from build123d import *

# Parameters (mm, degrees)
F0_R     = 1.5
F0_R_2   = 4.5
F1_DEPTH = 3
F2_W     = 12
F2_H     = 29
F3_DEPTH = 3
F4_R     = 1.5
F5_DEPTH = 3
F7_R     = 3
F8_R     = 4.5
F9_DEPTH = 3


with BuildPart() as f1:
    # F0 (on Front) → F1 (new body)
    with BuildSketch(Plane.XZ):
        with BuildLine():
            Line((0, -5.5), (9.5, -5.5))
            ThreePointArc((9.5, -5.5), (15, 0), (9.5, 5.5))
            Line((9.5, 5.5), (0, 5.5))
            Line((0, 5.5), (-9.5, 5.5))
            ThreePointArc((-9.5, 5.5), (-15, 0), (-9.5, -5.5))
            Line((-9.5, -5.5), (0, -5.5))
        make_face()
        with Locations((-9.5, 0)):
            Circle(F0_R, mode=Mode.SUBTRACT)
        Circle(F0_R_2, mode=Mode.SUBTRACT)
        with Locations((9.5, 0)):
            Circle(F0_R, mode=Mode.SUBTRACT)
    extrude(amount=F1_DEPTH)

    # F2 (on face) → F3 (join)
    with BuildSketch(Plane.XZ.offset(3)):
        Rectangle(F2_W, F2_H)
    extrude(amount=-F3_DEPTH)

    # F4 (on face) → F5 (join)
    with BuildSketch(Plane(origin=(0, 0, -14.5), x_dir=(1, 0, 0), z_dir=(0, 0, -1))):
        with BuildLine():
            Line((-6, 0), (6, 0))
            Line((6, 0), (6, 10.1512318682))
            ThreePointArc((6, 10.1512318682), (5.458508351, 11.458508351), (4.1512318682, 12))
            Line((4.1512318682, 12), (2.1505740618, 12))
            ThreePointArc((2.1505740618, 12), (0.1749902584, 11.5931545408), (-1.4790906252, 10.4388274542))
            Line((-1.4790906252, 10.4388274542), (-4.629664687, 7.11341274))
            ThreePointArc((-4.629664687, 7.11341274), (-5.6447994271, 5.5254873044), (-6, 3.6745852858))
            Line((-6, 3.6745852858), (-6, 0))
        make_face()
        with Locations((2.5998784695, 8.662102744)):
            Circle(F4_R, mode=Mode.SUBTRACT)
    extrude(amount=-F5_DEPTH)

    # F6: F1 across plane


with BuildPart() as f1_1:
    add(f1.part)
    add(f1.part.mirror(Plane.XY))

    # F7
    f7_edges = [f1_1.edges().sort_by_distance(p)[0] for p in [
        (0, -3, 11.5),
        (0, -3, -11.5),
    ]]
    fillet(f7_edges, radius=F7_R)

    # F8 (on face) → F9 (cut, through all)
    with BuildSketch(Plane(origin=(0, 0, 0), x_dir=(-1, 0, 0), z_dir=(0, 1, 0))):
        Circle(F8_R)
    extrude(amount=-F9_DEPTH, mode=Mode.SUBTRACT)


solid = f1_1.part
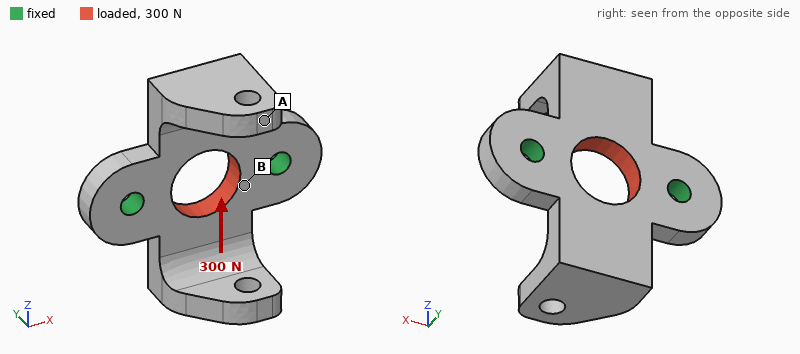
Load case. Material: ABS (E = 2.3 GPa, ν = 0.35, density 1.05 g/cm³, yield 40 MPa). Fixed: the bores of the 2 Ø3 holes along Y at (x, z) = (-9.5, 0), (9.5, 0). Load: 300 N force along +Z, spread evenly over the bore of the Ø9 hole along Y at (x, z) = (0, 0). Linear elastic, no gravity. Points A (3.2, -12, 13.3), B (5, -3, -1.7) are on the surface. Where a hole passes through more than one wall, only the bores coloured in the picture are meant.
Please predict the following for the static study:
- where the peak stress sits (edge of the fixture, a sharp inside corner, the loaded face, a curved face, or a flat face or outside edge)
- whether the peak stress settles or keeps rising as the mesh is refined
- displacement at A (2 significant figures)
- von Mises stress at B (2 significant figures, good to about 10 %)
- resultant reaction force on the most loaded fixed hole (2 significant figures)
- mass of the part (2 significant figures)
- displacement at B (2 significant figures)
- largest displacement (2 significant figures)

edge of the fixture
keeps rising
33 µm
6.4 MPa
150 N
1.9 g
29 µm
40 µm
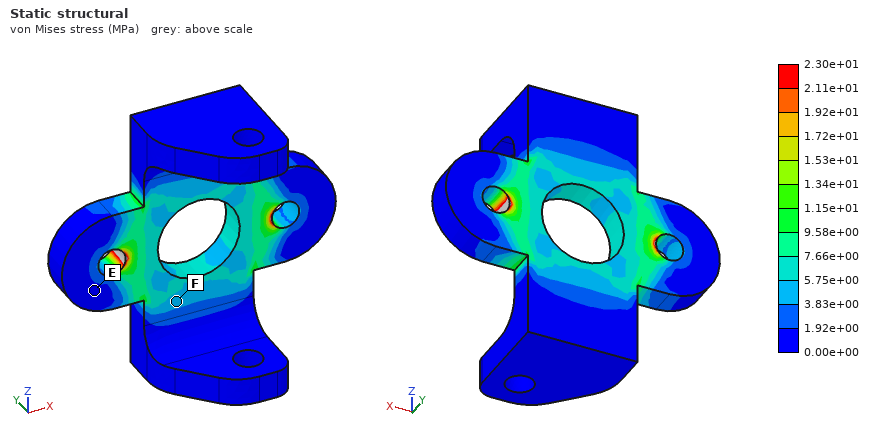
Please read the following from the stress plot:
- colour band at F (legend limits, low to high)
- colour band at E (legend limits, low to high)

3.83e+00 to 5.75e+00 MPa
0.00e+00 to 1.92e+00 MPa
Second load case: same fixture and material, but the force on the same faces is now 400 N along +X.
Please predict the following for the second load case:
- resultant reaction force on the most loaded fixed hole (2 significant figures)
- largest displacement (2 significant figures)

200 N
34 µm
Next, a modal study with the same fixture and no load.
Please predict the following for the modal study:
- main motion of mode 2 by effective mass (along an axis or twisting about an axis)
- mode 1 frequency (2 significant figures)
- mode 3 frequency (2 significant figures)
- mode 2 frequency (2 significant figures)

along Y
1700 Hz
4400 Hz
1800 Hz
